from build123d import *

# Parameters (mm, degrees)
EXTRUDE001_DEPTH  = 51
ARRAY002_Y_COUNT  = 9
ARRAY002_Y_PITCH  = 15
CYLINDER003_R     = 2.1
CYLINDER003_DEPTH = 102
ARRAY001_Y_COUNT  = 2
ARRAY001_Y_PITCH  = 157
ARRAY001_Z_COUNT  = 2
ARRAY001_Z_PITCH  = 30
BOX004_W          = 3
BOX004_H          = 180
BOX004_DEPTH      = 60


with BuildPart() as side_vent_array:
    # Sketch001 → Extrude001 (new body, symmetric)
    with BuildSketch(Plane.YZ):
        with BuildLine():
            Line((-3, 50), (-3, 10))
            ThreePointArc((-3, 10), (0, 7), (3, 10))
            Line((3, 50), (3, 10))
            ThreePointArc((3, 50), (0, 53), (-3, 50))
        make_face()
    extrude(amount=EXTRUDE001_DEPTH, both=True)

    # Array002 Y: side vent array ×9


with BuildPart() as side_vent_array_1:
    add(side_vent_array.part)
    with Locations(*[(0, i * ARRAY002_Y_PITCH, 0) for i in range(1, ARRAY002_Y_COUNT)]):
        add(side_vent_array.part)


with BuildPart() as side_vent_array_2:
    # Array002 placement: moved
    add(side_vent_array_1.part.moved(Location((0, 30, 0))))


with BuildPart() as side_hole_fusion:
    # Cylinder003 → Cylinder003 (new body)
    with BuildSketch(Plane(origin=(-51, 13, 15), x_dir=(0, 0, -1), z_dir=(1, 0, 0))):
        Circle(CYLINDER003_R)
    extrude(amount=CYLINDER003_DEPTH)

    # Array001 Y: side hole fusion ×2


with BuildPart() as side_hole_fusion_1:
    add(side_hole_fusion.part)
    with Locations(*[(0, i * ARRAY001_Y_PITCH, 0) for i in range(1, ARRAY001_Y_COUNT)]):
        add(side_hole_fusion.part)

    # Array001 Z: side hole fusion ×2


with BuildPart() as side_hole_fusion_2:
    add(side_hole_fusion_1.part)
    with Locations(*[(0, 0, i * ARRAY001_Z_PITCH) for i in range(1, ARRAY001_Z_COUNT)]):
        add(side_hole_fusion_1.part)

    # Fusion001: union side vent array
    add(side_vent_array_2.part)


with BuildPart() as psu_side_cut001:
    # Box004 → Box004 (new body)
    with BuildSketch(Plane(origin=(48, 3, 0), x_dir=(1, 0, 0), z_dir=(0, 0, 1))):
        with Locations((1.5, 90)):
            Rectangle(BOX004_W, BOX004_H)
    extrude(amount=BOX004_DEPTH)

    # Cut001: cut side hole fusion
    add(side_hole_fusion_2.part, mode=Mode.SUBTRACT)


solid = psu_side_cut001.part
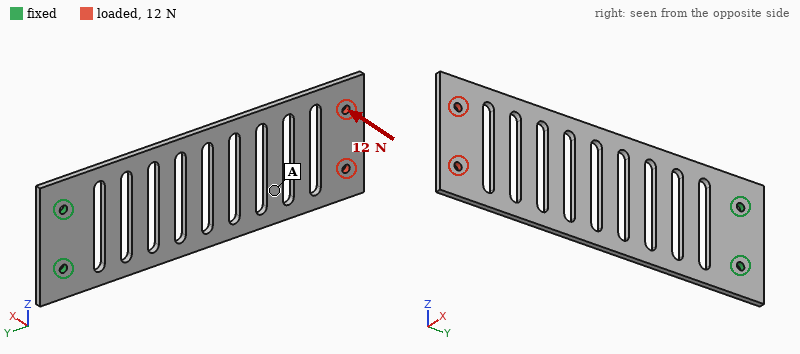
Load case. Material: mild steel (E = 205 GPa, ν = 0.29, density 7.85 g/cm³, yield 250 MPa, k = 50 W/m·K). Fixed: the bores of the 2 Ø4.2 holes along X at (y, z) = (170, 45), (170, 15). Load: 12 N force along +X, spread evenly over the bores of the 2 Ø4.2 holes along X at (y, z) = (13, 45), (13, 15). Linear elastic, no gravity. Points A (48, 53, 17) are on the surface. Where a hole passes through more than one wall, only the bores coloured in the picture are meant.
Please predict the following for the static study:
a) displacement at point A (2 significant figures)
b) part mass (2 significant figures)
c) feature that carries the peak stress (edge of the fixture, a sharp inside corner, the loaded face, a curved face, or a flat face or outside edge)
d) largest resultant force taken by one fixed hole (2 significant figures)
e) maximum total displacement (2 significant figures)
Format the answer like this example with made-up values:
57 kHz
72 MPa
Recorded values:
1.1 mm
200 g
a curved face
6.0 N
1.9 mm
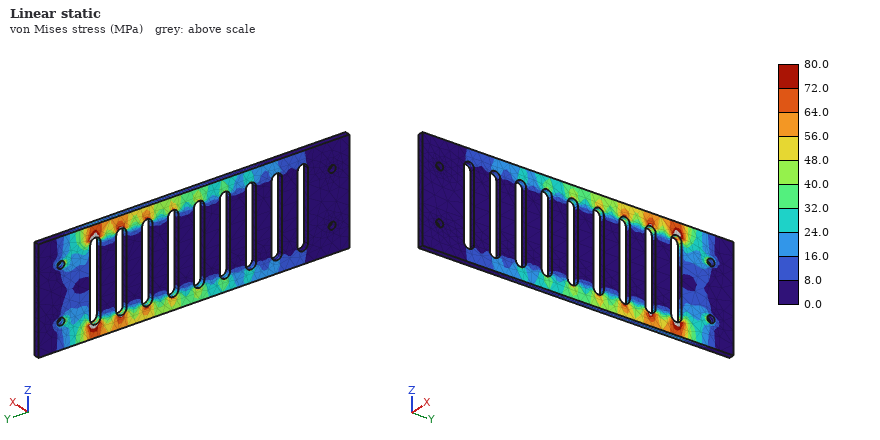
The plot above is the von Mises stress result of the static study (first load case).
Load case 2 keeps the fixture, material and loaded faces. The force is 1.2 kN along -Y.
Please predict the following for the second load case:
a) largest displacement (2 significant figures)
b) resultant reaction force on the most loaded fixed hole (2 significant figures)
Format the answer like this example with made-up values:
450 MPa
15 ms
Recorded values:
23 µm
610 N
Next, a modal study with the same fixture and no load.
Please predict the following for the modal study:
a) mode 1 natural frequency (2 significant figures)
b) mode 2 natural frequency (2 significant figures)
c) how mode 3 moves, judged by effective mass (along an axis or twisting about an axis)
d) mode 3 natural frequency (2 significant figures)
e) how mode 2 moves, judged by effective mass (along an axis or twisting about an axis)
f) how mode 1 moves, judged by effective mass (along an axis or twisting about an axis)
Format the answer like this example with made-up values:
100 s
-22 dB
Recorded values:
57 Hz
360 Hz
twisting about Y
430 Hz
along X
along X
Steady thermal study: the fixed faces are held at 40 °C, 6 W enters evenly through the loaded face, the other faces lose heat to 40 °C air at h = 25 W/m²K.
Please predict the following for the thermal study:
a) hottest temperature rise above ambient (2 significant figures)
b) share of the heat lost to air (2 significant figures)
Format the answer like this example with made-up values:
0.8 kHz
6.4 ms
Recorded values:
48 K
99 %
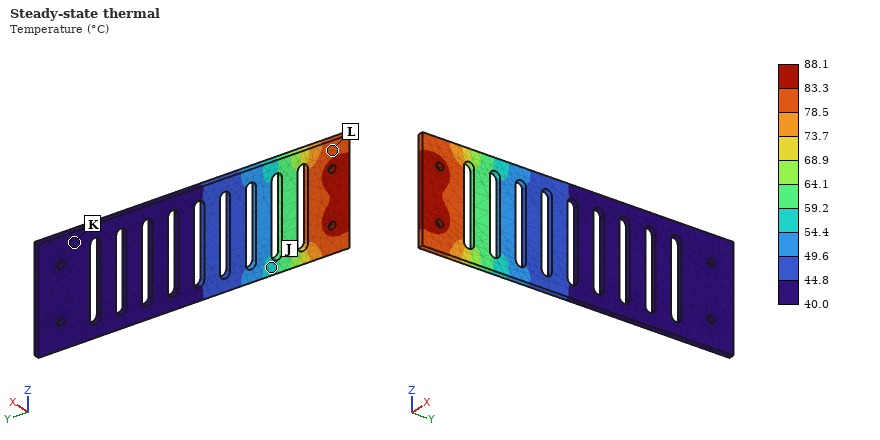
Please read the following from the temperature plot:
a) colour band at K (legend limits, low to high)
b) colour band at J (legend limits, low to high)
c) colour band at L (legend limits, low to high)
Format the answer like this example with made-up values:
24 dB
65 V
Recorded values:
40.0 to 44.8 °C
54.4 to 59.2 °C
78.5 to 83.3 °C
